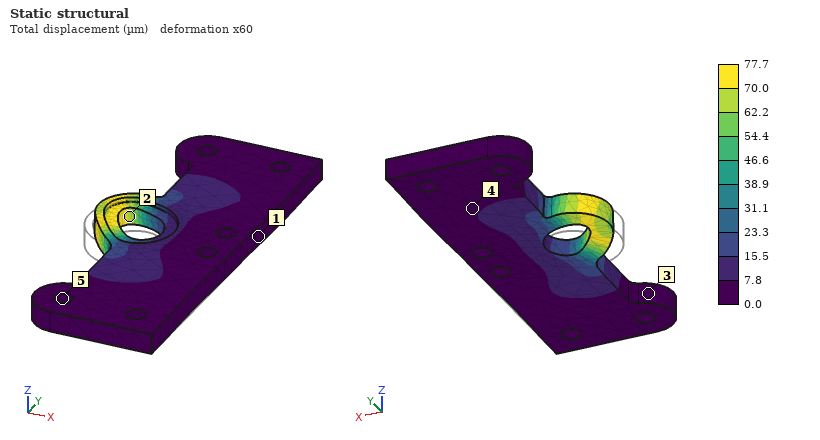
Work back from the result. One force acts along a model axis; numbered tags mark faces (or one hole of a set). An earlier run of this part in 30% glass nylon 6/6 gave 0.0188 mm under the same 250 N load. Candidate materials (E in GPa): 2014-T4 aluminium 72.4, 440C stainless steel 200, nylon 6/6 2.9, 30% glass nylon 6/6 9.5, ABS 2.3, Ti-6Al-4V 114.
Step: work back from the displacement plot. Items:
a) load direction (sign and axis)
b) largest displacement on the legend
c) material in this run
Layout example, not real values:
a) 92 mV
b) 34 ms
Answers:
a) +Y
b) 77.7 µm
c) ABS
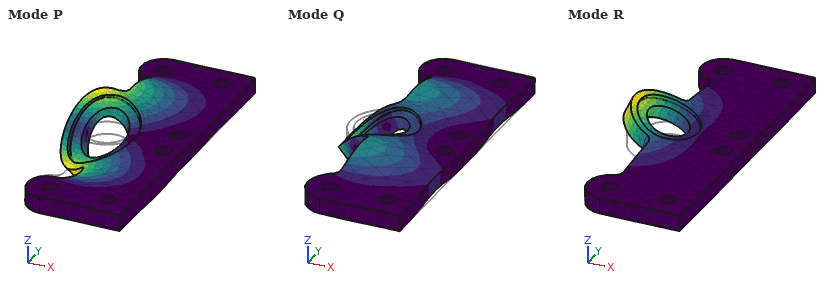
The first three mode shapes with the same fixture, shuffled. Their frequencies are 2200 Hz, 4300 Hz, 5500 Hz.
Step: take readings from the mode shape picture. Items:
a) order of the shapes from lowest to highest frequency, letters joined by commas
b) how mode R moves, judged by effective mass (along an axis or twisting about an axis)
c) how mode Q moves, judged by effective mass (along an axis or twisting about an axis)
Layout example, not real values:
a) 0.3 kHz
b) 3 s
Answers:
a) R, P, Q
b) along Z
c) along Z
